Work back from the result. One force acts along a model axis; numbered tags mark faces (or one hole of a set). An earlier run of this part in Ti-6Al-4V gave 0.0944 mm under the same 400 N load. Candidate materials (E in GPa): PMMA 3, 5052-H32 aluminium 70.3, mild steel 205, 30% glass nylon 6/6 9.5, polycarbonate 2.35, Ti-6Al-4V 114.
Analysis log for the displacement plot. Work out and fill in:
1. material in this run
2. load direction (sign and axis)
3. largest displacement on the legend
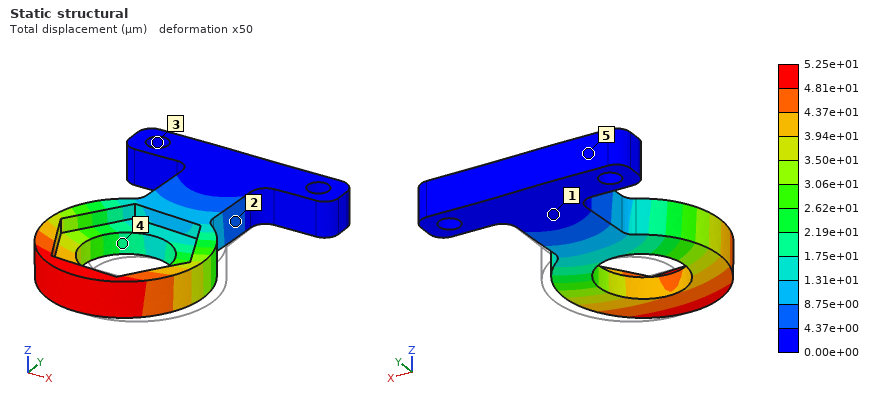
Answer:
mild steel
-X
5.25e+01 µm
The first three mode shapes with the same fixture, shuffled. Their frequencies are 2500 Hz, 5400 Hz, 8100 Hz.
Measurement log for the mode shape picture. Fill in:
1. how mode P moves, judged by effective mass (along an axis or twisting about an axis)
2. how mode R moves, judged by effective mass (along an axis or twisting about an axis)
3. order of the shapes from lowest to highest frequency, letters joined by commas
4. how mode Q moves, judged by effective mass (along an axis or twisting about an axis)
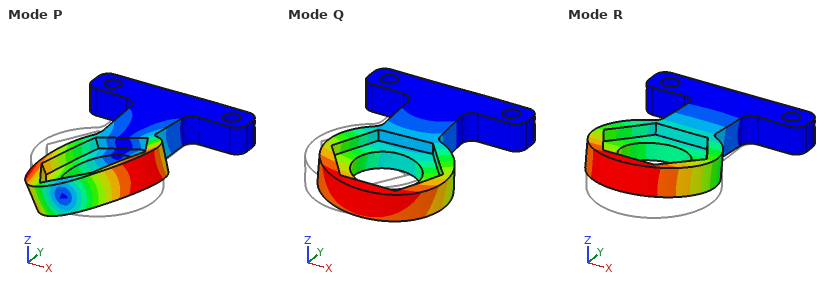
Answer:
twisting about Y
along Z
R, Q, P
along X
